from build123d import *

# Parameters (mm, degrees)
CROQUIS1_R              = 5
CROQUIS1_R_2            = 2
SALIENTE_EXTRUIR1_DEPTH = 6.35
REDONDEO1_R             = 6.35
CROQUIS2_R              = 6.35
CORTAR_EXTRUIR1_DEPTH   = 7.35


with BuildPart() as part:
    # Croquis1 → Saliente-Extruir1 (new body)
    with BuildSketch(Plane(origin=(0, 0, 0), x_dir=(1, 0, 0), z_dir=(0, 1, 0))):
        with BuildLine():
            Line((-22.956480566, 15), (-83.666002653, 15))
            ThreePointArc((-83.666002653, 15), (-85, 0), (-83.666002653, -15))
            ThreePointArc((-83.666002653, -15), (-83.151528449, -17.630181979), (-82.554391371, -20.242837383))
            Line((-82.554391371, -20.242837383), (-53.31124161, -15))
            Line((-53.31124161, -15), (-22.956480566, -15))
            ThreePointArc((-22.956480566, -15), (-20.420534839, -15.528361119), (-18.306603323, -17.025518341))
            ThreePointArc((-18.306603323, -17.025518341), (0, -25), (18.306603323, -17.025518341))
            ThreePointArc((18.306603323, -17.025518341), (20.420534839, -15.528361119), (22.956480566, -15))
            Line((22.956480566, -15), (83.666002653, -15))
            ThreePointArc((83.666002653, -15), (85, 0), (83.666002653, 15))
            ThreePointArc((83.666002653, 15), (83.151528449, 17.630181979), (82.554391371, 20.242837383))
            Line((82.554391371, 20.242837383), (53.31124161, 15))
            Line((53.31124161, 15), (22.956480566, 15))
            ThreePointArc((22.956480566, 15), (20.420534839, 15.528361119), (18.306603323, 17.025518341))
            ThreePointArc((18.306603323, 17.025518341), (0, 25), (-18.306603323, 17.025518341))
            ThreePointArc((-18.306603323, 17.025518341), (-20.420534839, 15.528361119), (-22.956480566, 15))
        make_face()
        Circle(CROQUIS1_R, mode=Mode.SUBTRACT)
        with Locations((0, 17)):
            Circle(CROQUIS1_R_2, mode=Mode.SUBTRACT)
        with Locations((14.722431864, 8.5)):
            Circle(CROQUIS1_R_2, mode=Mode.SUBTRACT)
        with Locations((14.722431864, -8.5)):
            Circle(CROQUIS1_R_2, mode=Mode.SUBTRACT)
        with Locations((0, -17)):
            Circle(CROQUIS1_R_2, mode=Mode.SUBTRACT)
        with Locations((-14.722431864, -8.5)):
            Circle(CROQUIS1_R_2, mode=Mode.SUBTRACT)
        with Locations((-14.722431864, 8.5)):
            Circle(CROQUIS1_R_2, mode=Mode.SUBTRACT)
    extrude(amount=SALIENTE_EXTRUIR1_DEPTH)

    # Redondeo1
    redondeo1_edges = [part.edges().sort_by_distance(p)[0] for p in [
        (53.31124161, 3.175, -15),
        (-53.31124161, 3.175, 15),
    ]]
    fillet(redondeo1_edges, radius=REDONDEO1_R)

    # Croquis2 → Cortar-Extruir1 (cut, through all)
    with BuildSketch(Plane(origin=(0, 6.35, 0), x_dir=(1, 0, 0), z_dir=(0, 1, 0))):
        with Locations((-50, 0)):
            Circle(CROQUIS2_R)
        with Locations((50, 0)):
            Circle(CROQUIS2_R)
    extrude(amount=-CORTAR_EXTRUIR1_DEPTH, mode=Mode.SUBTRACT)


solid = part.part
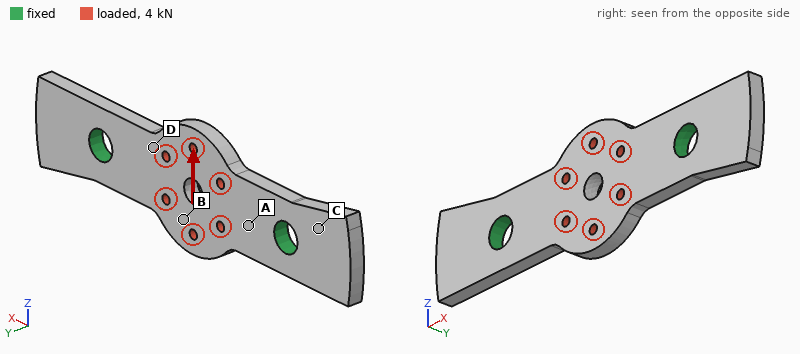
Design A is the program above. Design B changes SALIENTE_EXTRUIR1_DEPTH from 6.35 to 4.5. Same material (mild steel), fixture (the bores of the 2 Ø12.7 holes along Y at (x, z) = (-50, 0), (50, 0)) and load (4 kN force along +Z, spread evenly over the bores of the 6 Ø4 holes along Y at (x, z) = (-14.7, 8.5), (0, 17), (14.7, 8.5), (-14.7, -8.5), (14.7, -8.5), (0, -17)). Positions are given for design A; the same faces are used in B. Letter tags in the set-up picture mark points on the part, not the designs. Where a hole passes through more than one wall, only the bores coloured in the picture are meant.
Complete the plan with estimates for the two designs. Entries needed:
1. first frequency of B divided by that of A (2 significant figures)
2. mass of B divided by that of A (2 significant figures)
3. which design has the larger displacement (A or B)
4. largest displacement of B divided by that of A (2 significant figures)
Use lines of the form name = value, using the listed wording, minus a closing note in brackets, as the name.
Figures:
first frequency of B divided by that of A = 0.73
mass of B divided by that of A = 0.71
which design has the larger displacement = B
largest displacement of B divided by that of A = 1.4
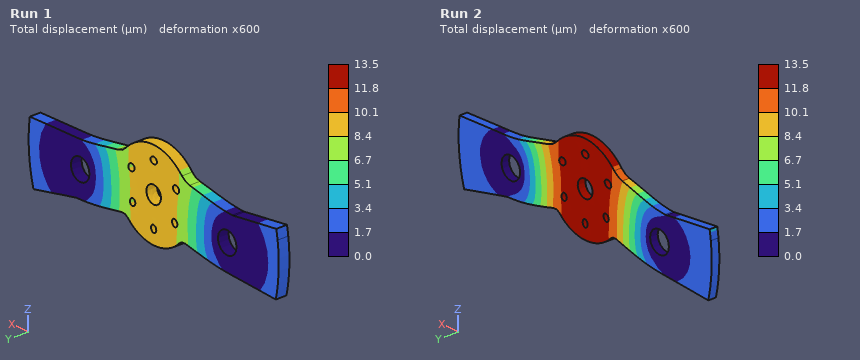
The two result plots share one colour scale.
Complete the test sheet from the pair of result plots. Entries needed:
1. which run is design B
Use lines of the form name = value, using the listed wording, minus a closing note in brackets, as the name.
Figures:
which run is design B = Run 2
